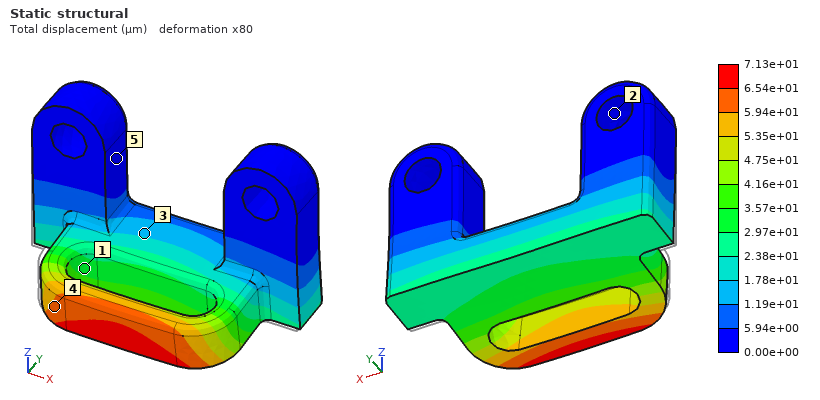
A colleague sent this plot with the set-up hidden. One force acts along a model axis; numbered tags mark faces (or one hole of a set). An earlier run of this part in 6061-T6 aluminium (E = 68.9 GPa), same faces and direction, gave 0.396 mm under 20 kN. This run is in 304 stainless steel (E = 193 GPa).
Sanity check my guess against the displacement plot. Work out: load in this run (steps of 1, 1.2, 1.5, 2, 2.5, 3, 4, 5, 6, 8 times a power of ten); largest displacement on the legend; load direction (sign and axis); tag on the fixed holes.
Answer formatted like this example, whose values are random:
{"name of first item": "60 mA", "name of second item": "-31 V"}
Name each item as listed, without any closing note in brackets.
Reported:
{"load in this run": "10 kN", "largest displacement on the legend": "7.13e+01 µm", "load direction": "-Z", "tag on the fixed holes": "2"}
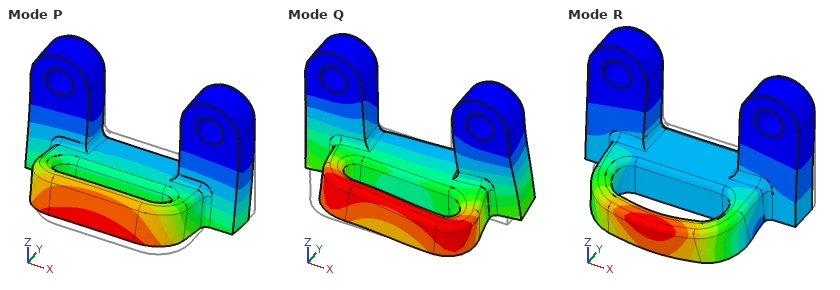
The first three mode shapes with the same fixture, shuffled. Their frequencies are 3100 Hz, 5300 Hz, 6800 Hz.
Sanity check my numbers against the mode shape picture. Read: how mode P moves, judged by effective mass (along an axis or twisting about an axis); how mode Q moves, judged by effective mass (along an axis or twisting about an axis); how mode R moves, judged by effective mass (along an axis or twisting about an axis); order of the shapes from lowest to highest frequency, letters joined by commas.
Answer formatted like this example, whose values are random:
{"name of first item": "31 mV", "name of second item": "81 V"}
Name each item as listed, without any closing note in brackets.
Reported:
{"how mode P moves, judged by effective mass": "along Y", "how mode Q moves, judged by effective mass": "along X", "how mode R moves, judged by effective mass": "along Y", "order of the shapes from lowest to highest frequency, letters joined by commas": "P, Q, R"}
